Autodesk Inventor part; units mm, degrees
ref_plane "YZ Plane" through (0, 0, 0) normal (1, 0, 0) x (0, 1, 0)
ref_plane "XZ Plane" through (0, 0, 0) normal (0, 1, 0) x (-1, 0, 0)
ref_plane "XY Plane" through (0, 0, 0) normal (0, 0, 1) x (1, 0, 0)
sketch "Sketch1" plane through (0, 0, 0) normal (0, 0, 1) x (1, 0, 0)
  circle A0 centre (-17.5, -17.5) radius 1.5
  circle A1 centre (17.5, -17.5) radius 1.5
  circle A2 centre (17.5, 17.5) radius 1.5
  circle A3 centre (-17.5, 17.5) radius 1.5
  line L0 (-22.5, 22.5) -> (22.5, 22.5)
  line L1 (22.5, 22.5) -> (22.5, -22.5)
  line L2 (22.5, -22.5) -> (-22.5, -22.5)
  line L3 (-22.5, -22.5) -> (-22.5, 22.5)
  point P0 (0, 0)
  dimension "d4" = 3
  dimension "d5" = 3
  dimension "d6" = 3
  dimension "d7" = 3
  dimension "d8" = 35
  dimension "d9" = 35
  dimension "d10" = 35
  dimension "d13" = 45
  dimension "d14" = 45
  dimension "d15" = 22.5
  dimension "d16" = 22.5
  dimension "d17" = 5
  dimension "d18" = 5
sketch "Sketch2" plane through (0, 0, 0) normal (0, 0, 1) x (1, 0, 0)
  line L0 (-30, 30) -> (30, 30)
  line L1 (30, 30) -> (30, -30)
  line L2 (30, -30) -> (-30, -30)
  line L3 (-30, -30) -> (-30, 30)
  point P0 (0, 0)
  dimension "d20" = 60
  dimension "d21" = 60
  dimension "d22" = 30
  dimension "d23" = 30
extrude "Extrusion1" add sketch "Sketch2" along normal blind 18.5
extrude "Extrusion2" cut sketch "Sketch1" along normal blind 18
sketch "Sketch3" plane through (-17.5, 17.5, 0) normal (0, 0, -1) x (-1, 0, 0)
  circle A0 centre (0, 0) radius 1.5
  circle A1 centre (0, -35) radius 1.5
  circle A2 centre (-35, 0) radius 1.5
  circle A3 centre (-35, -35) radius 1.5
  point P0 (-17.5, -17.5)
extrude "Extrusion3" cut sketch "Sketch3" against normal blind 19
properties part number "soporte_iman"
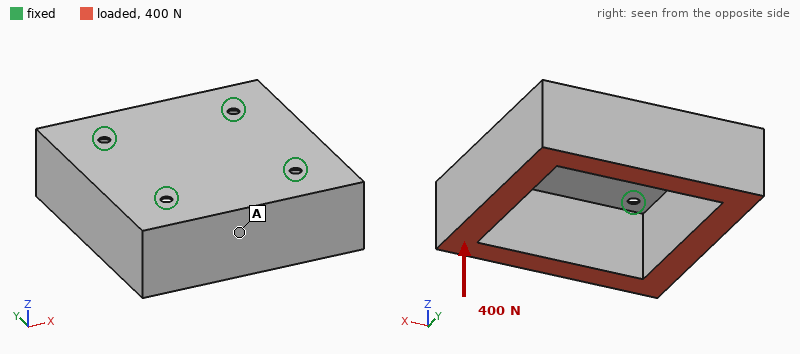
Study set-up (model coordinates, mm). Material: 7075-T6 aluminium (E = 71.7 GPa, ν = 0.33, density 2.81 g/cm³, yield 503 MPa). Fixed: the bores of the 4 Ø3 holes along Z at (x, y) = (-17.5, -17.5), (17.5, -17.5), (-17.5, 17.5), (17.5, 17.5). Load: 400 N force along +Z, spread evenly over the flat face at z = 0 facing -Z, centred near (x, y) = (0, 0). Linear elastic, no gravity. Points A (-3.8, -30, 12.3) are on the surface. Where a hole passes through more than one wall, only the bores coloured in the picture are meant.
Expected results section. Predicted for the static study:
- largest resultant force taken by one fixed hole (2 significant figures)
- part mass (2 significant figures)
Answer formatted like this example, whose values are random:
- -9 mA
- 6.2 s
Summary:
- 100 N
- 85 g
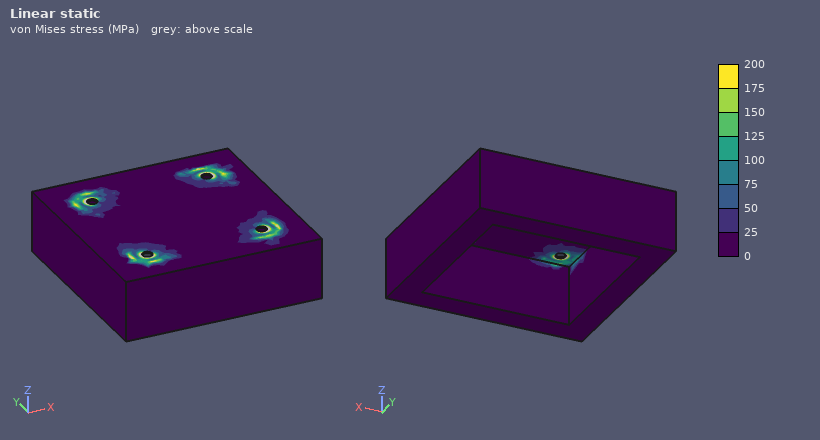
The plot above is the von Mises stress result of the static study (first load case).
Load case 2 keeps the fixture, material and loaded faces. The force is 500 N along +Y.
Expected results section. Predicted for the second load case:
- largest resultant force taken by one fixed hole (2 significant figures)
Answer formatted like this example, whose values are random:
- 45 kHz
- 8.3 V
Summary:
- 180 N
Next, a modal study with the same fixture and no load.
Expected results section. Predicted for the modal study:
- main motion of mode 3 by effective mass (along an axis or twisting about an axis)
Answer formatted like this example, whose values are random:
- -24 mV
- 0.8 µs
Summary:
- along Z
